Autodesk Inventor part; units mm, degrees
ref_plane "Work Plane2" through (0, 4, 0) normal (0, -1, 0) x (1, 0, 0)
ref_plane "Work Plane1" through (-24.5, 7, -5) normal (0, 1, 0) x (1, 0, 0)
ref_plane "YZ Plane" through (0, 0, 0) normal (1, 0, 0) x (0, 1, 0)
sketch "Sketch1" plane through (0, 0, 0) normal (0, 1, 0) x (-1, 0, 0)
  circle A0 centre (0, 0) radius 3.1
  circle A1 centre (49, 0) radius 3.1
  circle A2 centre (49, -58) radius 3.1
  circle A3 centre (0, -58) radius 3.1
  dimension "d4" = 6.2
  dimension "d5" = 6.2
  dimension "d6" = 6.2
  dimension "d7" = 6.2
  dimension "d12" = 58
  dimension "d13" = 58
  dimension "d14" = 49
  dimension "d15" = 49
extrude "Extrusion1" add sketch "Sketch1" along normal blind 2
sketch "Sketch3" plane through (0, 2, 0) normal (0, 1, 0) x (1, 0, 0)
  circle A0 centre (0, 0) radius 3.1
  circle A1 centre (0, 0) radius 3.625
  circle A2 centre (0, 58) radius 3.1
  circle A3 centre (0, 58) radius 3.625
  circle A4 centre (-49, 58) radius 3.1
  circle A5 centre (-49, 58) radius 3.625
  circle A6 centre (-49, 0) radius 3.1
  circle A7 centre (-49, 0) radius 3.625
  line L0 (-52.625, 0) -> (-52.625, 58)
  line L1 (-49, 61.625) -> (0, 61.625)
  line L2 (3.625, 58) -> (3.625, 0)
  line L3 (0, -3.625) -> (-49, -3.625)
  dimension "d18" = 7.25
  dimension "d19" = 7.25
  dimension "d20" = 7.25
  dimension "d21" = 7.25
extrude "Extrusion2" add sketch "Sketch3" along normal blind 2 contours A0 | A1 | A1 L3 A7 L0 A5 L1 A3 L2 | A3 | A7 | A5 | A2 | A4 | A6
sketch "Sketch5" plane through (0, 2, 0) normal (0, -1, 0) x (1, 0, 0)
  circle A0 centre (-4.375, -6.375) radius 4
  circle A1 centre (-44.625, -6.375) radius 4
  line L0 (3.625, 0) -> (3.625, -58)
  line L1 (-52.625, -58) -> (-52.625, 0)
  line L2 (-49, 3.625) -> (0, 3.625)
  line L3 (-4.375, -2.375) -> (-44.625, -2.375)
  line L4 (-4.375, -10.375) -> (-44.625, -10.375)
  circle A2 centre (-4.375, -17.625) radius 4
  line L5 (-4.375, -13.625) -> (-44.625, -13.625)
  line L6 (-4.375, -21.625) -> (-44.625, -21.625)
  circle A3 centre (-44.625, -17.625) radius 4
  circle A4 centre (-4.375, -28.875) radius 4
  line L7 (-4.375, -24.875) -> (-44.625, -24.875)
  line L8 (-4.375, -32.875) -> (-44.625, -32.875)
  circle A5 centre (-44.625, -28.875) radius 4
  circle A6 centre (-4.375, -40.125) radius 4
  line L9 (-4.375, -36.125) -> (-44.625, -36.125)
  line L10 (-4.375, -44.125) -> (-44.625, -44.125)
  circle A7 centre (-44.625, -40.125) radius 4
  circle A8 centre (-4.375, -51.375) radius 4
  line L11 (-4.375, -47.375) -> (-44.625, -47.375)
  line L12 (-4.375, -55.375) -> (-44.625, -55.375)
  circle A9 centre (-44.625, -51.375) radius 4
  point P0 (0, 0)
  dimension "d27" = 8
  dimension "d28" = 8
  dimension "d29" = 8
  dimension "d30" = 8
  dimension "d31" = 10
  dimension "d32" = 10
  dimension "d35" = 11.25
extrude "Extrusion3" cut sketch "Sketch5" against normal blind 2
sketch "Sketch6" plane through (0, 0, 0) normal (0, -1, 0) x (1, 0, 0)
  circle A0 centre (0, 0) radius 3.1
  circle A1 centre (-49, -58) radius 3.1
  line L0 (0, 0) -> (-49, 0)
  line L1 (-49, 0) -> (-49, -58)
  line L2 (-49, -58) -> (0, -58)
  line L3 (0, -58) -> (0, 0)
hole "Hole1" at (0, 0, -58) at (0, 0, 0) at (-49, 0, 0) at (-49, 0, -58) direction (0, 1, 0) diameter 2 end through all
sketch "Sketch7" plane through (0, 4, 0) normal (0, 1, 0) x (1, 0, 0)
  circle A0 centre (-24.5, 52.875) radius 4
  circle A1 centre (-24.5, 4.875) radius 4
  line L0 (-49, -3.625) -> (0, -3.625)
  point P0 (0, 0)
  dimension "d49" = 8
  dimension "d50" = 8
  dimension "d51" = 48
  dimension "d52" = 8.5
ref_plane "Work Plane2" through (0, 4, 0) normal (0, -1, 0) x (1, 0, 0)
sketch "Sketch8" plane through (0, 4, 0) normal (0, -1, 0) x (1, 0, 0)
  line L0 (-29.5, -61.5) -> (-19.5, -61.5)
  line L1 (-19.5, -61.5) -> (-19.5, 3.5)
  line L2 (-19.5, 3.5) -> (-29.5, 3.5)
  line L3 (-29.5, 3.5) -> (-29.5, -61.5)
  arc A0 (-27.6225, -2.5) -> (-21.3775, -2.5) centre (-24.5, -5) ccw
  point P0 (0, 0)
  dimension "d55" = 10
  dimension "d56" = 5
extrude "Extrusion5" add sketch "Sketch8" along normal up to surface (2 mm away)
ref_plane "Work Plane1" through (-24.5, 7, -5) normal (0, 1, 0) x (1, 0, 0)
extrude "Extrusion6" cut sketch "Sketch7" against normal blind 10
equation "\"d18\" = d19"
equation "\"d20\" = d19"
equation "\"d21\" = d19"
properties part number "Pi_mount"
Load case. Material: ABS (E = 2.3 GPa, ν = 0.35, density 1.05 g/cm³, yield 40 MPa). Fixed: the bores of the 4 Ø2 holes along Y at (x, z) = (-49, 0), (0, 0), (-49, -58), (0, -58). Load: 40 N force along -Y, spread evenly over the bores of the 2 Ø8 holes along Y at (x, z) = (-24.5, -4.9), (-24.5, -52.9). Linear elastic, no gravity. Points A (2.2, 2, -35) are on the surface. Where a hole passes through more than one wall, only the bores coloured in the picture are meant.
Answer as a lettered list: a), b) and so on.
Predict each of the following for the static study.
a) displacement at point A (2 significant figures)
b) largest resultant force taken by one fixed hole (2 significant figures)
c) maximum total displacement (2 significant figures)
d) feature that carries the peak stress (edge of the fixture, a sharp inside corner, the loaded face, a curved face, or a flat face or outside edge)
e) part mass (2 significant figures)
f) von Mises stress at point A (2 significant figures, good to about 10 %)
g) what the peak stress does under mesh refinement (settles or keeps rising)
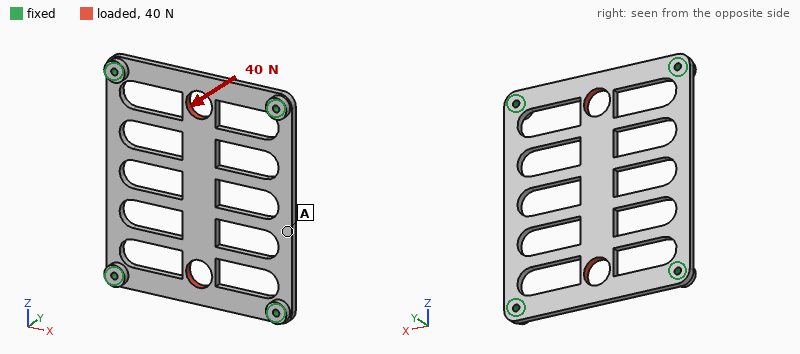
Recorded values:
a) 0.19 mm
b) 10 N
c) 0.85 mm
d) a sharp inside corner
e) 4.6 g
f) 1.9 MPa
g) keeps rising
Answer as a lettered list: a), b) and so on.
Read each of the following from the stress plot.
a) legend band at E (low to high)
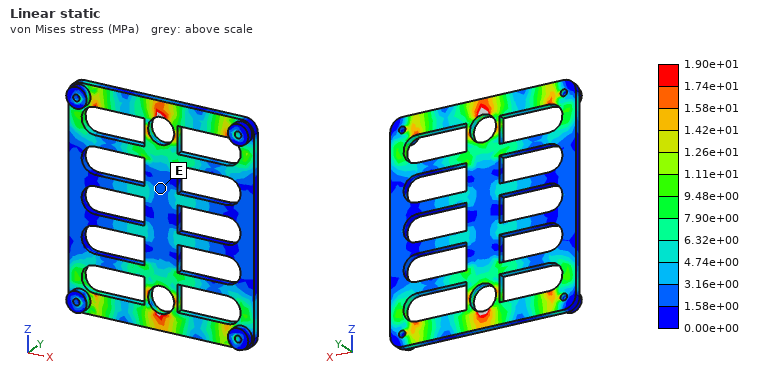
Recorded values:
a) 1.58e+00 to 3.16e+00 MPa
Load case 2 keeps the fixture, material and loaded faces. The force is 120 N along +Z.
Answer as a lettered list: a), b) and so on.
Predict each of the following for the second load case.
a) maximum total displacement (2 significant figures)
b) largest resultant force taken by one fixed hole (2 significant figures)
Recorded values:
a) 0.32 mm
b) 31 N
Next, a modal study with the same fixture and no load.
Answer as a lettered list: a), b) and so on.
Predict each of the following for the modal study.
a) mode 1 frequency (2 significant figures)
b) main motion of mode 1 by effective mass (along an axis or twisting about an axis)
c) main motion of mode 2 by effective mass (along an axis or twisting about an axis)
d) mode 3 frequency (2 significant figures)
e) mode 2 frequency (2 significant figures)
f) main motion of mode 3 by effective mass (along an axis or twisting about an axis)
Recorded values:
a) 590 Hz
b) along Y
c) twisting about Z
d) 1200 Hz
e) 970 Hz
f) twisting about X
